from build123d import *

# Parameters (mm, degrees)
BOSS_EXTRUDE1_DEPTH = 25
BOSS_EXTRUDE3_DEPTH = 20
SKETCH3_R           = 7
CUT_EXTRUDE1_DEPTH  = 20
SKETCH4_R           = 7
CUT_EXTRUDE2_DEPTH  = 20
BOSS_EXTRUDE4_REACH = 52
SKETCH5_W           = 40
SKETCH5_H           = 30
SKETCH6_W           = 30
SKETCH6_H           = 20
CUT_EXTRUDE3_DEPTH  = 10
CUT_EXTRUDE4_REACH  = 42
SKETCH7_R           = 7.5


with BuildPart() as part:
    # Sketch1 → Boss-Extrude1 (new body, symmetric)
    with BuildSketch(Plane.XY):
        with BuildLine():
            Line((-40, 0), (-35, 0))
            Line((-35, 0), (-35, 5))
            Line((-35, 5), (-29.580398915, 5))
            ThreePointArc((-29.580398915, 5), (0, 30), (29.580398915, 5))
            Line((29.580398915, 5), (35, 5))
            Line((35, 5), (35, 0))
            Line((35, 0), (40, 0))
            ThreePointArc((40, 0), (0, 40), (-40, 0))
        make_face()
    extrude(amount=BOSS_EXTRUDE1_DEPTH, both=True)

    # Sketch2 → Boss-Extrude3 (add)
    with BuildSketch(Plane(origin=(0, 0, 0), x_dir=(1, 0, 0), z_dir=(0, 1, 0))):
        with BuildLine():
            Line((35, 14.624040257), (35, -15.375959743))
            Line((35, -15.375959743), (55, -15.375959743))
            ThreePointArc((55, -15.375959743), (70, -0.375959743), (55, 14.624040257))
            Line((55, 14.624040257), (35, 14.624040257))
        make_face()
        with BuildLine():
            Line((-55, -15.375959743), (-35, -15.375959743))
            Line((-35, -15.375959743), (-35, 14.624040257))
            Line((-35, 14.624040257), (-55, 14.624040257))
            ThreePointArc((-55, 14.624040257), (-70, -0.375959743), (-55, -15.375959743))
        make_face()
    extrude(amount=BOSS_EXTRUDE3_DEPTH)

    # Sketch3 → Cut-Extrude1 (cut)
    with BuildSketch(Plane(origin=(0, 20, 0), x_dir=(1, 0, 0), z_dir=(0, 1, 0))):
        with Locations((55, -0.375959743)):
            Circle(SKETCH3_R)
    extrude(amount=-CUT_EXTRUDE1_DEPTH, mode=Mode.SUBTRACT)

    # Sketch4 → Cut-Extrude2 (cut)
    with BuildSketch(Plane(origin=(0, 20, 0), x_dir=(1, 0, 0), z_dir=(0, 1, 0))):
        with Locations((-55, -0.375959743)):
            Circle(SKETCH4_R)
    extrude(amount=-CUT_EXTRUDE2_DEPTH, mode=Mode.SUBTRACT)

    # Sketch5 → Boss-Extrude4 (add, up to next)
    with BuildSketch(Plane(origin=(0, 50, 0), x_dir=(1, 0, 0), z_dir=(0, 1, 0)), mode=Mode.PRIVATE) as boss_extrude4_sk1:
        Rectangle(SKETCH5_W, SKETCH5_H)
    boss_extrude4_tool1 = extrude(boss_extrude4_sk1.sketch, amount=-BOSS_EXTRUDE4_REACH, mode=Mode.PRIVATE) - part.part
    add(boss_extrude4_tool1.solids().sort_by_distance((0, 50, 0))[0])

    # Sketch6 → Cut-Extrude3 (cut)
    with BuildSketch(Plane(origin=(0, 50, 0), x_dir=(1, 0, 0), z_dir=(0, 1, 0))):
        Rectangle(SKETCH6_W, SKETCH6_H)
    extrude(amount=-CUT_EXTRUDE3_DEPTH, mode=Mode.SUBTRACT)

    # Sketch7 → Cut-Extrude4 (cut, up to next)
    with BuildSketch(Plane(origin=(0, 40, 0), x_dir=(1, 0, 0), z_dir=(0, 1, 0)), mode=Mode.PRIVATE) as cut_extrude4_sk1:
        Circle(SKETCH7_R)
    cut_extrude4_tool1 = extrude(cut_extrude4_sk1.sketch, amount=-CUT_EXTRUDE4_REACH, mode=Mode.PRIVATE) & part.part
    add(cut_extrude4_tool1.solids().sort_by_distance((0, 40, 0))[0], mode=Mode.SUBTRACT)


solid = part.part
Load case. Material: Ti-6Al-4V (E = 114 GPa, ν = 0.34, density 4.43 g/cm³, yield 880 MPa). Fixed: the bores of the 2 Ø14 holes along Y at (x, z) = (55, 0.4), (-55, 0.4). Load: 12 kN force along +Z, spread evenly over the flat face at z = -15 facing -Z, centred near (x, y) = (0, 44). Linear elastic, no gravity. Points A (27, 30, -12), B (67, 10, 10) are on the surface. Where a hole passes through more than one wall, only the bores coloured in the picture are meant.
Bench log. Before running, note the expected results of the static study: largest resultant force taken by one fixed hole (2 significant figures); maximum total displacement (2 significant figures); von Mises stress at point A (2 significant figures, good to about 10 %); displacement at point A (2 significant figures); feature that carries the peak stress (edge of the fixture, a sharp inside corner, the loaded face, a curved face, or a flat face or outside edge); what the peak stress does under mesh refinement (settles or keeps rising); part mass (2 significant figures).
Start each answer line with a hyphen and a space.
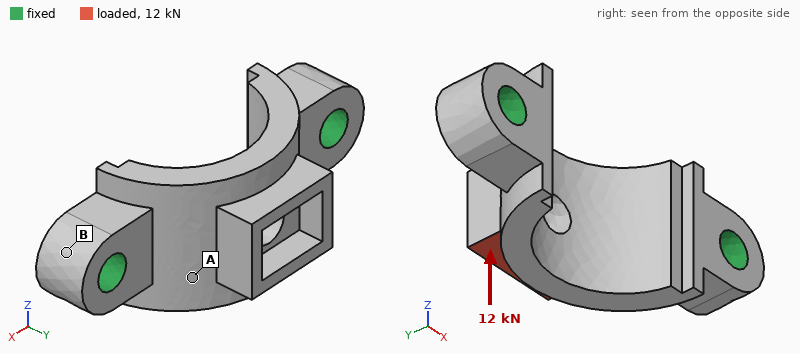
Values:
- 6.0 kN
- 0.19 mm
- 55 MPa
- 0.070 mm
- edge of the fixture
- keeps rising
- 380 g
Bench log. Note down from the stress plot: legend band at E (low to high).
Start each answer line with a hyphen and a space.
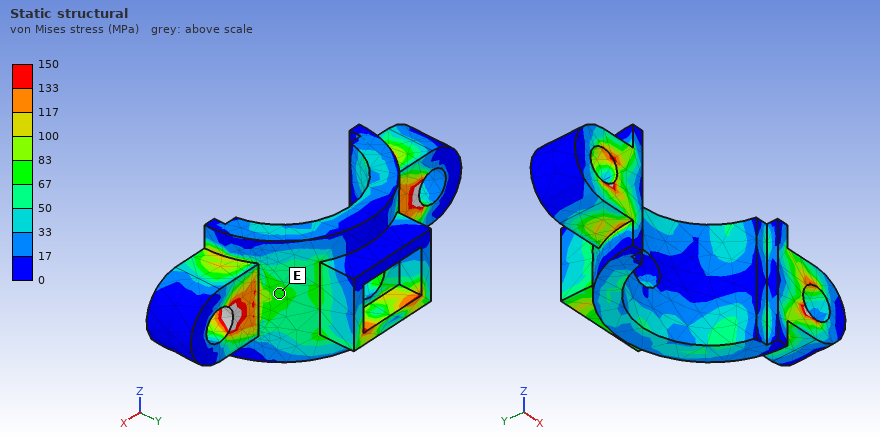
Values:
- 67 to 83 MPa
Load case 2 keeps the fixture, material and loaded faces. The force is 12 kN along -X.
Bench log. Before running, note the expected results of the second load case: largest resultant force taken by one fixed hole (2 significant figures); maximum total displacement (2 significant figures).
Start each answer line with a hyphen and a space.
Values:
- 7.9 kN
- 37 µm
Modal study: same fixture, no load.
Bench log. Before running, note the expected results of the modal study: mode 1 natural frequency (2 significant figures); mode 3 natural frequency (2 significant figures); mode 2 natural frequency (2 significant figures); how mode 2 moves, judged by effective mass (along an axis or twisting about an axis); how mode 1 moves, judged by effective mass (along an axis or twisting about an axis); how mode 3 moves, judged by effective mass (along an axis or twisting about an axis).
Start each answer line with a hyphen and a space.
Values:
- 4700 Hz
- 10 kHz
- 10000 Hz
- along Y
- along Z
- along X
